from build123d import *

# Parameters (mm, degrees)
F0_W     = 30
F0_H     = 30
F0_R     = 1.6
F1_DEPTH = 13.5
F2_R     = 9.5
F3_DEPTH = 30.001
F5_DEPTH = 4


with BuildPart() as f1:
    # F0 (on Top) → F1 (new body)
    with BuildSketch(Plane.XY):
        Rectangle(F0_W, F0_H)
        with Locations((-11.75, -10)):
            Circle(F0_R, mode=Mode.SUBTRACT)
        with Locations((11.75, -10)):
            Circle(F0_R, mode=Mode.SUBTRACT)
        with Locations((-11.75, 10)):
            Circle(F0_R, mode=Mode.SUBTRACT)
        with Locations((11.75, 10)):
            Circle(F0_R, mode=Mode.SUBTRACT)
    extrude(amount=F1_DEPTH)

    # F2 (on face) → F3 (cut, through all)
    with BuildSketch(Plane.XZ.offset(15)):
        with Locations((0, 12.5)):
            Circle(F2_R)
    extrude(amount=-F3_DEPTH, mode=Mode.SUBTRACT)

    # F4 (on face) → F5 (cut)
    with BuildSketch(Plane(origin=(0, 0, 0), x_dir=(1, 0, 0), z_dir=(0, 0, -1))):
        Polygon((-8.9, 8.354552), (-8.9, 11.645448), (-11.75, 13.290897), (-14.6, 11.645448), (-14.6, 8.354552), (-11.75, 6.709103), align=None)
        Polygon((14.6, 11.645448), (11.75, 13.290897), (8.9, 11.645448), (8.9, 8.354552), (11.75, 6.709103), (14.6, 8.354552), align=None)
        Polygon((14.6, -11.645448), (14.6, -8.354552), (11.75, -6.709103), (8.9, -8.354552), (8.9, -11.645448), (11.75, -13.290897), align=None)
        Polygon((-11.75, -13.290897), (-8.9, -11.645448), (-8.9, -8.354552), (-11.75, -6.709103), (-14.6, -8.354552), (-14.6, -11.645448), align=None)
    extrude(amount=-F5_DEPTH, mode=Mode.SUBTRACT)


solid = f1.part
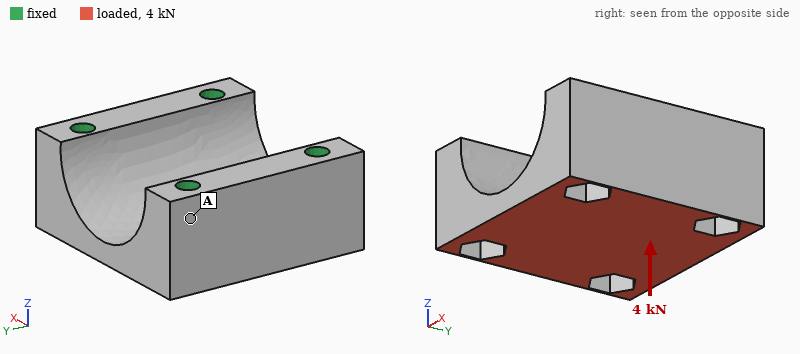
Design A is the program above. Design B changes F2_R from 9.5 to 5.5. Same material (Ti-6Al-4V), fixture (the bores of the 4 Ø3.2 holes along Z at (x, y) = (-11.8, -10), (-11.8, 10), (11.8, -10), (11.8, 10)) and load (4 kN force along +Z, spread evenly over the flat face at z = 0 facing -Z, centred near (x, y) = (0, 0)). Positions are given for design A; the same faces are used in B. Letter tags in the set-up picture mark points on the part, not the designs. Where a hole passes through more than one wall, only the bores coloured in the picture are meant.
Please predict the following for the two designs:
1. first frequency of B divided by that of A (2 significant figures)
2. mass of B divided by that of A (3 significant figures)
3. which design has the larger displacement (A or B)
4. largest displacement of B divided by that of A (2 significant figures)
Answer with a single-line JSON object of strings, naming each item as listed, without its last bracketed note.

{"first frequency of B divided by that of A": "0.98", "mass of B divided by that of A": "1.47", "which design has the larger displacement": "A", "largest displacement of B divided by that of A": "0.46"}
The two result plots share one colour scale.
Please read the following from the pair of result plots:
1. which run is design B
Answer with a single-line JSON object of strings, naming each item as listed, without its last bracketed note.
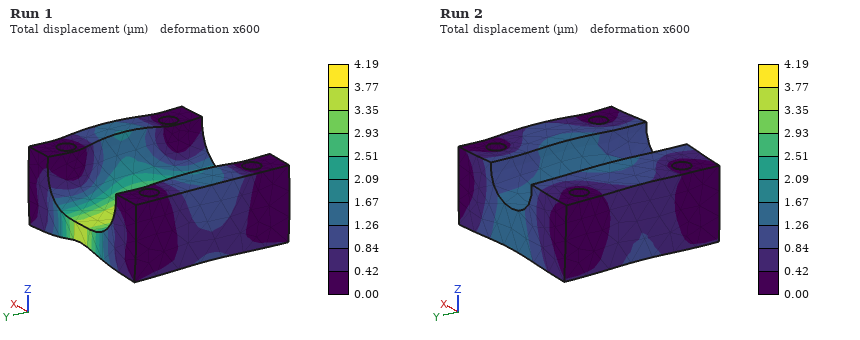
{"which run is design B": "Run 2"}
